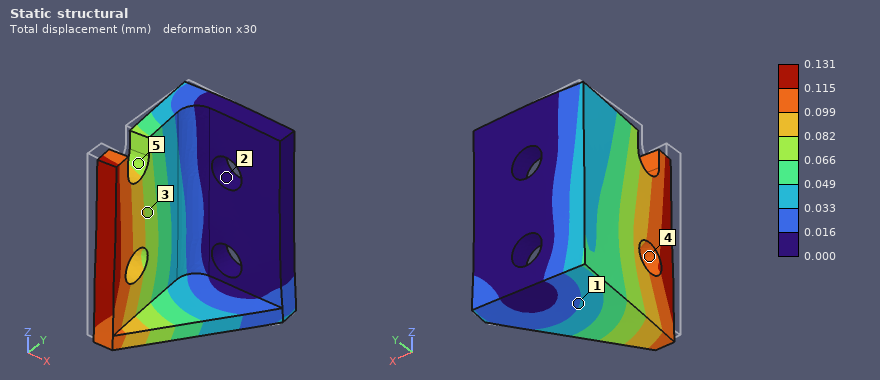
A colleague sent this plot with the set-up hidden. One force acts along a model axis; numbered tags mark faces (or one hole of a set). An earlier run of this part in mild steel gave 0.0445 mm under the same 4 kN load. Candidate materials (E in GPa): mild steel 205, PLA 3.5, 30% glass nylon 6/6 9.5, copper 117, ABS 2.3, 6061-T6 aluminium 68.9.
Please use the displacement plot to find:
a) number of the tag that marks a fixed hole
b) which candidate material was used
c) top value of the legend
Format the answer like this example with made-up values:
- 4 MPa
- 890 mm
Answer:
- 2
- 6061-T6 aluminium
- 0.131 mm
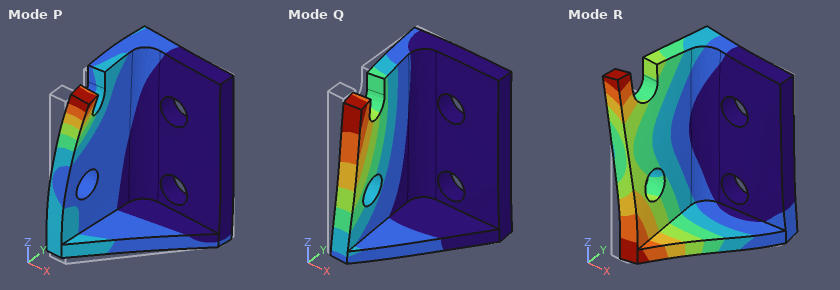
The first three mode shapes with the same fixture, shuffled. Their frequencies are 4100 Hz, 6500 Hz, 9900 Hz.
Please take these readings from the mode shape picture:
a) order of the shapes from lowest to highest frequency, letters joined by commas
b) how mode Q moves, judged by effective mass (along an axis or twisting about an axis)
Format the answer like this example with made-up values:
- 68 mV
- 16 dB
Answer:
- Q, R, P
- along X
